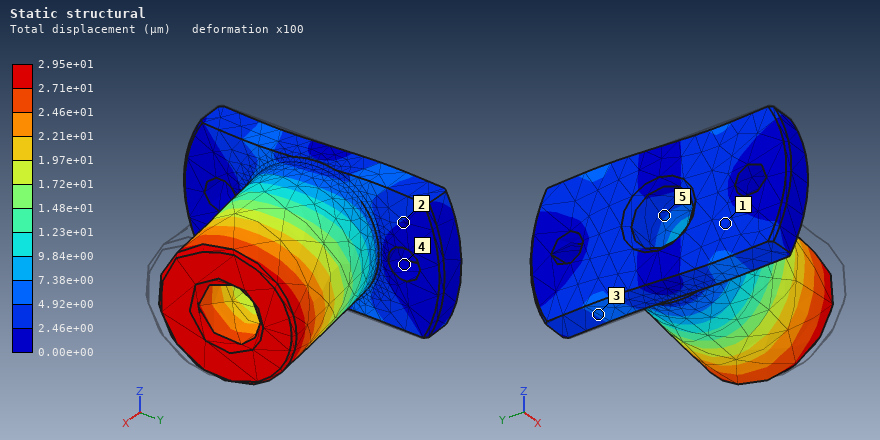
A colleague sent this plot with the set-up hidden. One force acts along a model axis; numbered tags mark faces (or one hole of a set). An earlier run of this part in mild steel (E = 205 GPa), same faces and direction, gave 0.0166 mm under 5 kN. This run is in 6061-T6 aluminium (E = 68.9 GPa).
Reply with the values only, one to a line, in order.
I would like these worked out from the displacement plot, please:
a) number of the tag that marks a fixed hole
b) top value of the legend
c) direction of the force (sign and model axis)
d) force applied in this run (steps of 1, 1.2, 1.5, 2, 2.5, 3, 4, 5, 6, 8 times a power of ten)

4
2.95e+01 µm
+Y
3 kN
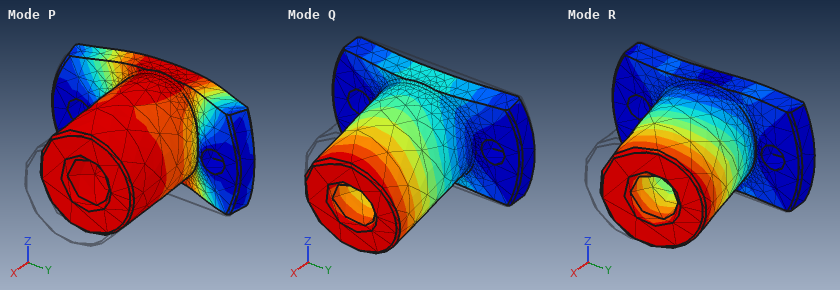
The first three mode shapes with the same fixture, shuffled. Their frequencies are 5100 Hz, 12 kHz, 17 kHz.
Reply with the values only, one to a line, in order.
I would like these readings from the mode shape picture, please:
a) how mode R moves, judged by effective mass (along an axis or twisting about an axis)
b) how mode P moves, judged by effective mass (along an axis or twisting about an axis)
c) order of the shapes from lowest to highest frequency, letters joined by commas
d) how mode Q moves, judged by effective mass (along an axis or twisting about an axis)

along Y
along X
Q, R, P
along Z
